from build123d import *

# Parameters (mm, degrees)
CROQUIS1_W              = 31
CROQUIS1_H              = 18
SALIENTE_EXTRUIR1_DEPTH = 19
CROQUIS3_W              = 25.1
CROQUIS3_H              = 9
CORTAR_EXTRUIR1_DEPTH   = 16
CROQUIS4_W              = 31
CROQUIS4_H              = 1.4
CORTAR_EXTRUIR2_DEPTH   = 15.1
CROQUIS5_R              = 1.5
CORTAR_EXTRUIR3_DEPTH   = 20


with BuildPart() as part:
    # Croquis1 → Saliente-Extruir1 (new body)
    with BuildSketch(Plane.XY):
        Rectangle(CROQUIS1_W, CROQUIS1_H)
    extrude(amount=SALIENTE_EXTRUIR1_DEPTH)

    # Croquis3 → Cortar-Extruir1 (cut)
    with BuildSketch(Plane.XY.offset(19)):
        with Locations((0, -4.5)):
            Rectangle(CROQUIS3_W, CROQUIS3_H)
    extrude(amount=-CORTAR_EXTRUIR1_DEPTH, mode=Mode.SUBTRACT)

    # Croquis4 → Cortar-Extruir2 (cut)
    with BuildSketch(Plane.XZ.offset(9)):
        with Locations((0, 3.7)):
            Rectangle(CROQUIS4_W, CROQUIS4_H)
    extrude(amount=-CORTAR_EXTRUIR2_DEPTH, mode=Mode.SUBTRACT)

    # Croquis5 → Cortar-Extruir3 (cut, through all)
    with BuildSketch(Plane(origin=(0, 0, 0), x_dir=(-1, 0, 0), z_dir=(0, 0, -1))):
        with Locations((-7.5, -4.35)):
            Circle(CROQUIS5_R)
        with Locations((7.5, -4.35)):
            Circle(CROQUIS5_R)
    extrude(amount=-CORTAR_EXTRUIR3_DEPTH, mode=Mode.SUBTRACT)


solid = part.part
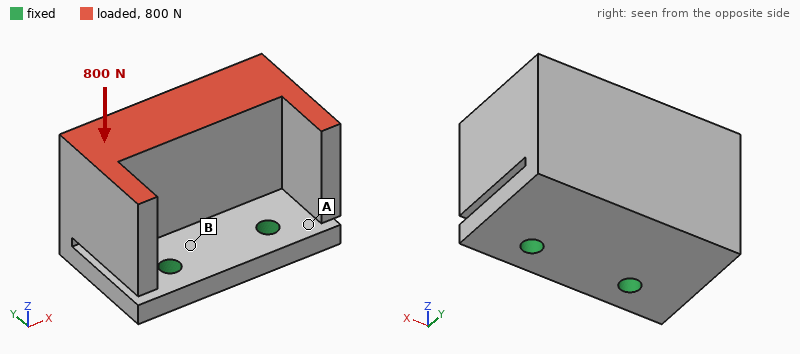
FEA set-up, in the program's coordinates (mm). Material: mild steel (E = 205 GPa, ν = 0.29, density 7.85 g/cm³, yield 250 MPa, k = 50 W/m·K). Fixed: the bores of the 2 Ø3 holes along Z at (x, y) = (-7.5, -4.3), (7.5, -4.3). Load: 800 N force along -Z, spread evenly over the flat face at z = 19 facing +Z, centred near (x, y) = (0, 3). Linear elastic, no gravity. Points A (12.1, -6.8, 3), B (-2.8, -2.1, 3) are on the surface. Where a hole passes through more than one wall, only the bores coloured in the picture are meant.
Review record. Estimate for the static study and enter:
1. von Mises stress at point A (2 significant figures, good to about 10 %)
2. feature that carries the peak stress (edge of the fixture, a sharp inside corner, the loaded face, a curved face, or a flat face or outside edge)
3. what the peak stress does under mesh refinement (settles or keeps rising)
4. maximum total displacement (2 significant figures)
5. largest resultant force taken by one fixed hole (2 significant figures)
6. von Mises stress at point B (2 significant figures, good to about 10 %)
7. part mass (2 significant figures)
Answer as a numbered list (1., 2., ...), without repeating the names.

1. 24 MPa
2. edge of the fixture
3. keeps rising
4. 18 µm
5. 400 N
6. 55 MPa
7. 52 g
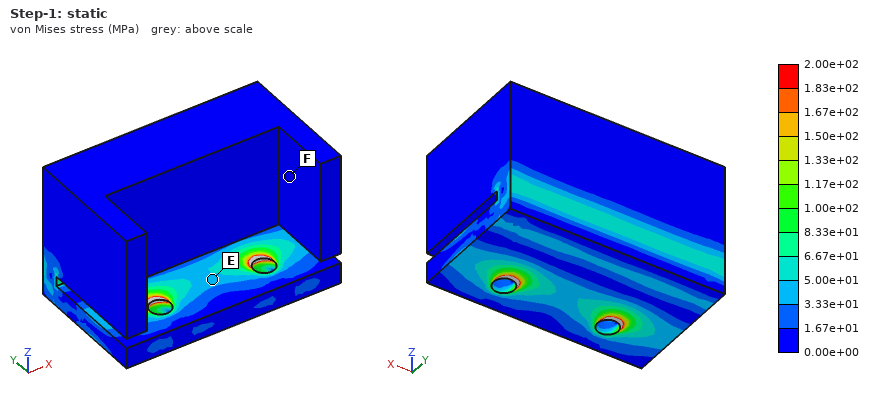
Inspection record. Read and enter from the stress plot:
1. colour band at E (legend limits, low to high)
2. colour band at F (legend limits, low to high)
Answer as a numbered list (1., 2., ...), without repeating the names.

1. 3.33e+01 to 5.00e+01 MPa
2. 0.00e+00 to 1.67e+01 MPa
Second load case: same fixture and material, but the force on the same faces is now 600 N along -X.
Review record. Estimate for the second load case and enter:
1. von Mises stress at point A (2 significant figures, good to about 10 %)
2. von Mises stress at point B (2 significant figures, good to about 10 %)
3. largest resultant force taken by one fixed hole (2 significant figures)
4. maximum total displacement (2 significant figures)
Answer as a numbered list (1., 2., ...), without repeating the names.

1. 50 MPa
2. 66 MPa
3. 660 N
4. 55 µm
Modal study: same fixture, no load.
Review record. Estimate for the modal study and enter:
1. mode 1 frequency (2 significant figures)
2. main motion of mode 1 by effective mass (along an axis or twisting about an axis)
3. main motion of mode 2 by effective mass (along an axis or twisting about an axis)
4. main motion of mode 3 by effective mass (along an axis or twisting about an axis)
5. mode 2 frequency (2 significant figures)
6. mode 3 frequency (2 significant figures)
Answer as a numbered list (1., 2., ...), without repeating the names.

1. 2200 Hz
2. along Y
3. along X
4. along Z
5. 3700 Hz
6. 5600 Hz
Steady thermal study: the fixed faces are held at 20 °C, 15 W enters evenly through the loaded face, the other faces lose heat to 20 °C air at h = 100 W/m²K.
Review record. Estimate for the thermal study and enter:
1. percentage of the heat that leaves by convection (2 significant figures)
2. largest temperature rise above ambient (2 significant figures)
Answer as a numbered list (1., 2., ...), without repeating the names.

1. 51 %
2. 39 K
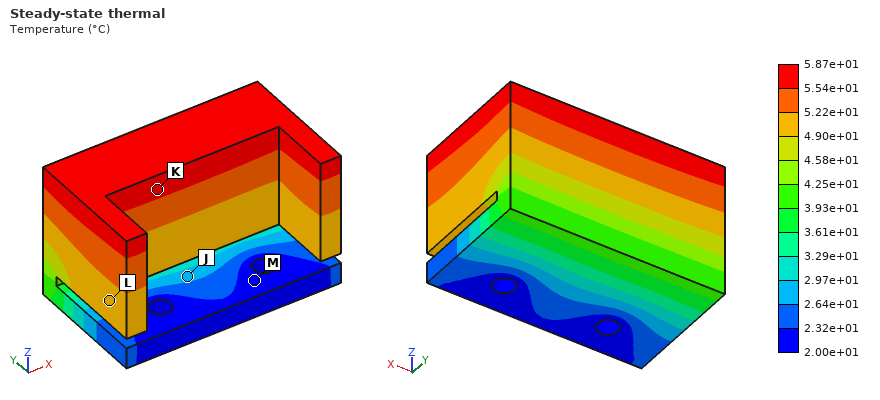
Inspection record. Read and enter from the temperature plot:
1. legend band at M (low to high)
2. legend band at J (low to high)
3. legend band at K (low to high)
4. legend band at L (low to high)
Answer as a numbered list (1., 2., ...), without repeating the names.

1. 2.00e+01 to 2.32e+01 °C
2. 2.64e+01 to 2.97e+01 °C
3. 5.54e+01 to 5.87e+01 °C
4. 4.90e+01 to 5.22e+01 °C
